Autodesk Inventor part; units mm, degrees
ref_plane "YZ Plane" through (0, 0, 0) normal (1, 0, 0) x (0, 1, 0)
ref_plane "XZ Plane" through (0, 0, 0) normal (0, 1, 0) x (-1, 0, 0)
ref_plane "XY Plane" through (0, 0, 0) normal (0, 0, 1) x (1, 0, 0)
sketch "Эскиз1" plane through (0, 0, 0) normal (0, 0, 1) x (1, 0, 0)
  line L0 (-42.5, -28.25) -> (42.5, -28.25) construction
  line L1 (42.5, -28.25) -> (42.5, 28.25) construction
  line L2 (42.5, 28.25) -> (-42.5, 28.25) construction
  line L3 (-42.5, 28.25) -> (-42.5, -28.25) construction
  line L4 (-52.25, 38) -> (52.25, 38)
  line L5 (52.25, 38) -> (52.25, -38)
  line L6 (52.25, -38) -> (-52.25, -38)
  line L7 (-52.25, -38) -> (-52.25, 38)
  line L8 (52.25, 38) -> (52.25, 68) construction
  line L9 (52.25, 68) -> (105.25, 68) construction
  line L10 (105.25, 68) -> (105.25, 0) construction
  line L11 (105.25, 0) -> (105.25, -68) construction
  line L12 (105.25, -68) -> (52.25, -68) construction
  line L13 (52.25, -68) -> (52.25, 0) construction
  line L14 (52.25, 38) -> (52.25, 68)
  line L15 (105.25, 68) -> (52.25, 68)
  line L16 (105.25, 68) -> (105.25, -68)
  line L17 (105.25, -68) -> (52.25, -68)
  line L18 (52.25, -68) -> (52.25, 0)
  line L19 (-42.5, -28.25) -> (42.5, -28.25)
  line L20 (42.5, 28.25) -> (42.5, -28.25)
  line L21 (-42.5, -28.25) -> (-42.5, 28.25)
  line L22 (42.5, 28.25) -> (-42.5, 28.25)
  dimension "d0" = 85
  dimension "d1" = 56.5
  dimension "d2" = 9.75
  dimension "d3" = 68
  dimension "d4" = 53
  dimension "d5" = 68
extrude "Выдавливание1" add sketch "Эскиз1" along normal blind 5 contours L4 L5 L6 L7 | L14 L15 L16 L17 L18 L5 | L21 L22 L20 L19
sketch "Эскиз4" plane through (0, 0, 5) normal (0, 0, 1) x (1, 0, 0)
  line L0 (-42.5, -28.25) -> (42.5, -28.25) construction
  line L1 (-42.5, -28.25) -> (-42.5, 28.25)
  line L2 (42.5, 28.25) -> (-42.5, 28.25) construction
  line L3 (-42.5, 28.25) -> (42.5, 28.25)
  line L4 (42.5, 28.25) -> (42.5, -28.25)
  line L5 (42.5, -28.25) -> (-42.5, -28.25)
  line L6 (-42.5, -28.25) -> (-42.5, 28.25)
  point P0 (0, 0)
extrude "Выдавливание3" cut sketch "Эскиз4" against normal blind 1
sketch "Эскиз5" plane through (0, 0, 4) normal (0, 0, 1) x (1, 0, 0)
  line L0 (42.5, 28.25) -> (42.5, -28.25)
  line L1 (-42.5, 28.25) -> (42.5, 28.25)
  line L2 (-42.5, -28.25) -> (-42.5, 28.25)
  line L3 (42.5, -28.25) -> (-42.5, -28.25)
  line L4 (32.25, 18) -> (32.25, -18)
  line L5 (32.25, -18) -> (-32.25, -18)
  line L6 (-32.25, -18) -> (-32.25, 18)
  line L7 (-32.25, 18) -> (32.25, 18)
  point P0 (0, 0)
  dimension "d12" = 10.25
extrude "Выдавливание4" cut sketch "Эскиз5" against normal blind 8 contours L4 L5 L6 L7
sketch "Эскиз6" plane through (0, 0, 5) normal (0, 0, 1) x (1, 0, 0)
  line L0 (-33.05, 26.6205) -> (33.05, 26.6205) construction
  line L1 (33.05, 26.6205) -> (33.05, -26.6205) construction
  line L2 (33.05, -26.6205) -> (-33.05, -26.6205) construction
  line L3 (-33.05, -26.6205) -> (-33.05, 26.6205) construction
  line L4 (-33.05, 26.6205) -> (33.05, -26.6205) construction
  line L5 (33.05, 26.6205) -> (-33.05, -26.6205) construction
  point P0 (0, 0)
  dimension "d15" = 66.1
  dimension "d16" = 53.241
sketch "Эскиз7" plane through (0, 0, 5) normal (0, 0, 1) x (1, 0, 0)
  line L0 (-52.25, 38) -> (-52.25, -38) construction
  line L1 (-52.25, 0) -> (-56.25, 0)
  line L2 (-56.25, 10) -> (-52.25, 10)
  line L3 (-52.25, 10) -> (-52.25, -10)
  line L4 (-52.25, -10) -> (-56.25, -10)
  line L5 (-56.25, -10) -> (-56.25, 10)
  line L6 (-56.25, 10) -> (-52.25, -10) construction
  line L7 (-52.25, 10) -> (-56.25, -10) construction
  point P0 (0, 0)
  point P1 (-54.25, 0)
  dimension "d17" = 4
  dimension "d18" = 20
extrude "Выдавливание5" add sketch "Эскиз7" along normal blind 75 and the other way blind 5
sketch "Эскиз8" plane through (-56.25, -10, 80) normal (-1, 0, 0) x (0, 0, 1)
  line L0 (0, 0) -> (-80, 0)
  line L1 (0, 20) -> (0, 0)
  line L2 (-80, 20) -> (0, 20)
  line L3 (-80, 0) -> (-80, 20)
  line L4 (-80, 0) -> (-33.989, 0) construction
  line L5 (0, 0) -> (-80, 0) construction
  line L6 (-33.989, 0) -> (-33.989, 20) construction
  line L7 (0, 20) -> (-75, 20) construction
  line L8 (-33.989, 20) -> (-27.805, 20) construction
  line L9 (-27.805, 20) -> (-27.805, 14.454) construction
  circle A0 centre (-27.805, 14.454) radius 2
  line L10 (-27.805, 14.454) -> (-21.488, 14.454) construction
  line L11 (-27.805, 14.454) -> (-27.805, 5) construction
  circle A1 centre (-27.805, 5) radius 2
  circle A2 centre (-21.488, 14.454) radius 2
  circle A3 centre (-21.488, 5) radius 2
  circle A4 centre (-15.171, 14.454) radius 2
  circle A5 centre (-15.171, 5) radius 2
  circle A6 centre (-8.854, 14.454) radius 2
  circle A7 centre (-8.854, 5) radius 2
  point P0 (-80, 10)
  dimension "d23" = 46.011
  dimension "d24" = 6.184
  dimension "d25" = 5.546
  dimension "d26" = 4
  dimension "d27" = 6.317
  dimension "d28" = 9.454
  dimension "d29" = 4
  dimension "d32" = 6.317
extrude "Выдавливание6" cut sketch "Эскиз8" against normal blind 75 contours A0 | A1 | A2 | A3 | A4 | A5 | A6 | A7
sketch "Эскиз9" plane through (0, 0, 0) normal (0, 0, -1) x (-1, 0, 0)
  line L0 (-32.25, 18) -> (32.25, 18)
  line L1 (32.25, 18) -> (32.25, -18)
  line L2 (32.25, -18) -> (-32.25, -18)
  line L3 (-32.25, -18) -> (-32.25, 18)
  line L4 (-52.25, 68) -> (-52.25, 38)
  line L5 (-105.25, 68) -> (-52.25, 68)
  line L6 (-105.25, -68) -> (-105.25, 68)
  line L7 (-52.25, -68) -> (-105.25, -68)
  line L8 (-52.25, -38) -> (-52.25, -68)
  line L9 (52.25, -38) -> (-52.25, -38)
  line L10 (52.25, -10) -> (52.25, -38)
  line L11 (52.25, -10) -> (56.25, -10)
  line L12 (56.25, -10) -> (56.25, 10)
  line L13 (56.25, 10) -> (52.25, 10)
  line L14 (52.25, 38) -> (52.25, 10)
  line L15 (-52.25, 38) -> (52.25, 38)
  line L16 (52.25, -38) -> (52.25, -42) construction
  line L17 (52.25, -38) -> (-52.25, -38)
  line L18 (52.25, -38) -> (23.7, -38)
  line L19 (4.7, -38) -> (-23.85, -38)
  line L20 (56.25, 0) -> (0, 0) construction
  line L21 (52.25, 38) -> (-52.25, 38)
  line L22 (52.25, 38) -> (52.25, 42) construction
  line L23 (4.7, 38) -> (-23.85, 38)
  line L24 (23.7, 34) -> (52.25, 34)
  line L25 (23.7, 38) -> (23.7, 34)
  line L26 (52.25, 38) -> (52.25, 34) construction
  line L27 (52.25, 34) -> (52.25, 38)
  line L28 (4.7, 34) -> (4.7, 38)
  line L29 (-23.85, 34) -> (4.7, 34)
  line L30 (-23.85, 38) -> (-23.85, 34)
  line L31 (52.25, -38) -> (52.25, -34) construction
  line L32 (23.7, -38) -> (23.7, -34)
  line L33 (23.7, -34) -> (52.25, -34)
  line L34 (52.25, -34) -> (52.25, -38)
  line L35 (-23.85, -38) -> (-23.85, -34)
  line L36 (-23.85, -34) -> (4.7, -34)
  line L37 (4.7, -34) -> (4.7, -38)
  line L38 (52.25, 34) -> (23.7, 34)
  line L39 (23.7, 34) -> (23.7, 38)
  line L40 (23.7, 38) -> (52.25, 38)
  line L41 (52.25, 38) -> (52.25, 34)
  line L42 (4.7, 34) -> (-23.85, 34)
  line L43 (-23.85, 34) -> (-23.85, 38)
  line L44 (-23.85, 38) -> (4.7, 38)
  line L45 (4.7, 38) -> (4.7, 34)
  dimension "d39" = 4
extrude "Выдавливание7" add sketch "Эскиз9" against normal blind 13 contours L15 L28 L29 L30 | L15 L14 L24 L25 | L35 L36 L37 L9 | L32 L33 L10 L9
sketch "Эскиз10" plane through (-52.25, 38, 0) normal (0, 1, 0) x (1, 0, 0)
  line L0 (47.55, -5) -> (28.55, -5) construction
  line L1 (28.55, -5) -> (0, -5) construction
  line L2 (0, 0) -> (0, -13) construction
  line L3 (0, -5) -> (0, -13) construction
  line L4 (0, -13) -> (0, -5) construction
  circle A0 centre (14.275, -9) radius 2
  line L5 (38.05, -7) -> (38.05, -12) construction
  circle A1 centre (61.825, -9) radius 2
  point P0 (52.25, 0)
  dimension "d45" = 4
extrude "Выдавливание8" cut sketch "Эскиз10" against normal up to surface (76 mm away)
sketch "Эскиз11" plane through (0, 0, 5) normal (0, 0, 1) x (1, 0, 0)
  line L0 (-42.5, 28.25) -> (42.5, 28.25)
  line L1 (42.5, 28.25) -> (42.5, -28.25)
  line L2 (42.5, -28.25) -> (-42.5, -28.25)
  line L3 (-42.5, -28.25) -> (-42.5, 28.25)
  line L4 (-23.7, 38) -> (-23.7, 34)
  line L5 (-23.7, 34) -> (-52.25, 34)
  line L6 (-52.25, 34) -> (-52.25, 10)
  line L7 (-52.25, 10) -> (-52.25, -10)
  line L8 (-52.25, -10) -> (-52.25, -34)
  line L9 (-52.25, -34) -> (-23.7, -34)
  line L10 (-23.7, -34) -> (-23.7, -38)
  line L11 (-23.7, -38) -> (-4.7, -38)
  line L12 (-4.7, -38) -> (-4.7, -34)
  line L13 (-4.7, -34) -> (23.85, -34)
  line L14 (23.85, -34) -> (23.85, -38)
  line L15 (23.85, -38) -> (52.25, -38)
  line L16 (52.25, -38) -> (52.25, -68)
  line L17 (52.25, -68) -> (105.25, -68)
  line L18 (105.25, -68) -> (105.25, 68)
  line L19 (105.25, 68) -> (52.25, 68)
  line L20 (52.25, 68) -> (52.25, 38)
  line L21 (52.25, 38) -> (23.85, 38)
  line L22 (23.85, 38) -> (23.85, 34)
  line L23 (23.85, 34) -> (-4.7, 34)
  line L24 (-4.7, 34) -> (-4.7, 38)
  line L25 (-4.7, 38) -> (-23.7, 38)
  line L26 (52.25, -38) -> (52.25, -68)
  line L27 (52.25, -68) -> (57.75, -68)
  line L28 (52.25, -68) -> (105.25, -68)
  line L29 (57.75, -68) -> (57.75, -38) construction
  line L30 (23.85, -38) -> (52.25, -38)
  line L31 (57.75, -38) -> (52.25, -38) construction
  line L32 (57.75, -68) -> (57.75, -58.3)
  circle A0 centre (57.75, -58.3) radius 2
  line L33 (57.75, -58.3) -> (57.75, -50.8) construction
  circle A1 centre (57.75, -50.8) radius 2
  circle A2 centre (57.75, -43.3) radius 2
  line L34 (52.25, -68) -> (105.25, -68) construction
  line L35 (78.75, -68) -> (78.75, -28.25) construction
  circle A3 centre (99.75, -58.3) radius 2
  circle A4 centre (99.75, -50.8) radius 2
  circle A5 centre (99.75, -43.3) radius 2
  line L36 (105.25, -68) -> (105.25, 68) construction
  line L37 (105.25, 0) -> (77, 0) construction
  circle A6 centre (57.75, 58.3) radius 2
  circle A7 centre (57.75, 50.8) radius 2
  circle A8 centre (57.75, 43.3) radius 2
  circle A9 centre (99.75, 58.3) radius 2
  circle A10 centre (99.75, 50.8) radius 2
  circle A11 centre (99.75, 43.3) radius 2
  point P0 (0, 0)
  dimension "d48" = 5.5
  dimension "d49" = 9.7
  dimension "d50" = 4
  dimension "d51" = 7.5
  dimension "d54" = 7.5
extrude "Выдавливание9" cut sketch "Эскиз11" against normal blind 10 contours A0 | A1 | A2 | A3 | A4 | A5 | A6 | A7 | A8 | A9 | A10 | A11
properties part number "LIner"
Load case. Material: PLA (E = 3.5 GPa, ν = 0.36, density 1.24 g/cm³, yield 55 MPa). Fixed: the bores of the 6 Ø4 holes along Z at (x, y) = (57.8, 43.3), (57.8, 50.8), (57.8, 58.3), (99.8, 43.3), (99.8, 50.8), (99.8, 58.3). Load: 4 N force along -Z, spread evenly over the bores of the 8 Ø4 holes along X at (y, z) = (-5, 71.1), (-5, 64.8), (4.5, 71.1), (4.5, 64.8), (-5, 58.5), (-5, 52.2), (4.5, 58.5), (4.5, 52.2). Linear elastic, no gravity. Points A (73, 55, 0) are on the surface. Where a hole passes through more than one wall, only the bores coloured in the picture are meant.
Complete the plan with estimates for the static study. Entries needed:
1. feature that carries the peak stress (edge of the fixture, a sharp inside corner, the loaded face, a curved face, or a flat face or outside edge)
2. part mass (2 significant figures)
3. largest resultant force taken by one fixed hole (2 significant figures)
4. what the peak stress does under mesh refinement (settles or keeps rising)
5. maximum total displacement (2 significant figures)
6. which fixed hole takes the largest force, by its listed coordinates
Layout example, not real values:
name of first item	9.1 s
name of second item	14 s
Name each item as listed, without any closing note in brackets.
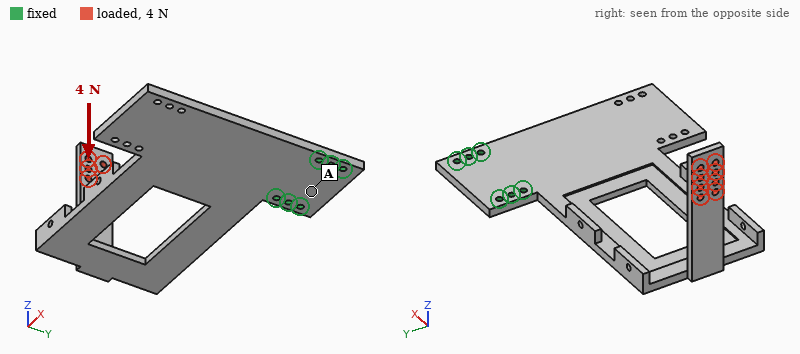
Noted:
feature that carries the peak stress	edge of the fixture
part mass	87 g
largest resultant force taken by one fixed hole	19 N
what the peak stress does under mesh refinement	keeps rising
maximum total displacement	2.3 mm
which fixed hole takes the largest force, by its listed coordinates	(57.8, 43.3)
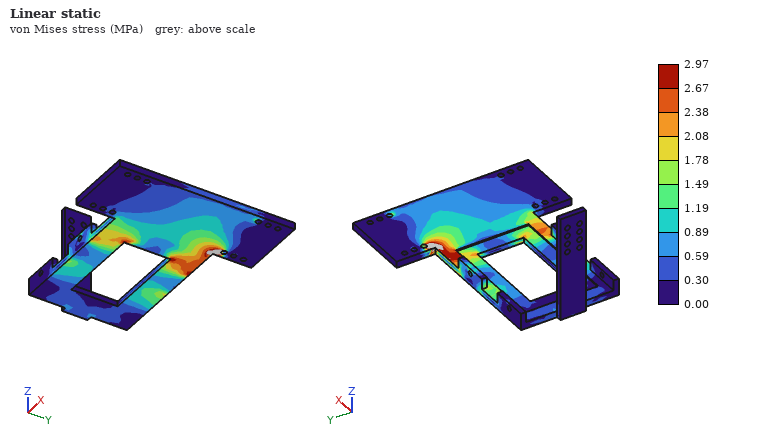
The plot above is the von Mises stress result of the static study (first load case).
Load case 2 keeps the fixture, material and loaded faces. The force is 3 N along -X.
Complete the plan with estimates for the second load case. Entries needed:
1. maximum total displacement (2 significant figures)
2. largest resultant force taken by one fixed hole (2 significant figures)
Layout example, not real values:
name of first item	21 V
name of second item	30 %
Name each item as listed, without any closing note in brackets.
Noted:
maximum total displacement	2.1 mm
largest resultant force taken by one fixed hole	5.6 N
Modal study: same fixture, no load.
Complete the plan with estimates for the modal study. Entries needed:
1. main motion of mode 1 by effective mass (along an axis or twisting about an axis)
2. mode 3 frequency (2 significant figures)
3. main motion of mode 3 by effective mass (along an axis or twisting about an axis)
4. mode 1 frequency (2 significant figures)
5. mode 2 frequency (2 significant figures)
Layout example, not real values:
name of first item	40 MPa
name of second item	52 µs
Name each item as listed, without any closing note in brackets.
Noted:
main motion of mode 1 by effective mass	along Z
mode 3 frequency	160 Hz
main motion of mode 3 by effective mass	along Z
mode 1 frequency	54 Hz
mode 2 frequency	93 Hz
